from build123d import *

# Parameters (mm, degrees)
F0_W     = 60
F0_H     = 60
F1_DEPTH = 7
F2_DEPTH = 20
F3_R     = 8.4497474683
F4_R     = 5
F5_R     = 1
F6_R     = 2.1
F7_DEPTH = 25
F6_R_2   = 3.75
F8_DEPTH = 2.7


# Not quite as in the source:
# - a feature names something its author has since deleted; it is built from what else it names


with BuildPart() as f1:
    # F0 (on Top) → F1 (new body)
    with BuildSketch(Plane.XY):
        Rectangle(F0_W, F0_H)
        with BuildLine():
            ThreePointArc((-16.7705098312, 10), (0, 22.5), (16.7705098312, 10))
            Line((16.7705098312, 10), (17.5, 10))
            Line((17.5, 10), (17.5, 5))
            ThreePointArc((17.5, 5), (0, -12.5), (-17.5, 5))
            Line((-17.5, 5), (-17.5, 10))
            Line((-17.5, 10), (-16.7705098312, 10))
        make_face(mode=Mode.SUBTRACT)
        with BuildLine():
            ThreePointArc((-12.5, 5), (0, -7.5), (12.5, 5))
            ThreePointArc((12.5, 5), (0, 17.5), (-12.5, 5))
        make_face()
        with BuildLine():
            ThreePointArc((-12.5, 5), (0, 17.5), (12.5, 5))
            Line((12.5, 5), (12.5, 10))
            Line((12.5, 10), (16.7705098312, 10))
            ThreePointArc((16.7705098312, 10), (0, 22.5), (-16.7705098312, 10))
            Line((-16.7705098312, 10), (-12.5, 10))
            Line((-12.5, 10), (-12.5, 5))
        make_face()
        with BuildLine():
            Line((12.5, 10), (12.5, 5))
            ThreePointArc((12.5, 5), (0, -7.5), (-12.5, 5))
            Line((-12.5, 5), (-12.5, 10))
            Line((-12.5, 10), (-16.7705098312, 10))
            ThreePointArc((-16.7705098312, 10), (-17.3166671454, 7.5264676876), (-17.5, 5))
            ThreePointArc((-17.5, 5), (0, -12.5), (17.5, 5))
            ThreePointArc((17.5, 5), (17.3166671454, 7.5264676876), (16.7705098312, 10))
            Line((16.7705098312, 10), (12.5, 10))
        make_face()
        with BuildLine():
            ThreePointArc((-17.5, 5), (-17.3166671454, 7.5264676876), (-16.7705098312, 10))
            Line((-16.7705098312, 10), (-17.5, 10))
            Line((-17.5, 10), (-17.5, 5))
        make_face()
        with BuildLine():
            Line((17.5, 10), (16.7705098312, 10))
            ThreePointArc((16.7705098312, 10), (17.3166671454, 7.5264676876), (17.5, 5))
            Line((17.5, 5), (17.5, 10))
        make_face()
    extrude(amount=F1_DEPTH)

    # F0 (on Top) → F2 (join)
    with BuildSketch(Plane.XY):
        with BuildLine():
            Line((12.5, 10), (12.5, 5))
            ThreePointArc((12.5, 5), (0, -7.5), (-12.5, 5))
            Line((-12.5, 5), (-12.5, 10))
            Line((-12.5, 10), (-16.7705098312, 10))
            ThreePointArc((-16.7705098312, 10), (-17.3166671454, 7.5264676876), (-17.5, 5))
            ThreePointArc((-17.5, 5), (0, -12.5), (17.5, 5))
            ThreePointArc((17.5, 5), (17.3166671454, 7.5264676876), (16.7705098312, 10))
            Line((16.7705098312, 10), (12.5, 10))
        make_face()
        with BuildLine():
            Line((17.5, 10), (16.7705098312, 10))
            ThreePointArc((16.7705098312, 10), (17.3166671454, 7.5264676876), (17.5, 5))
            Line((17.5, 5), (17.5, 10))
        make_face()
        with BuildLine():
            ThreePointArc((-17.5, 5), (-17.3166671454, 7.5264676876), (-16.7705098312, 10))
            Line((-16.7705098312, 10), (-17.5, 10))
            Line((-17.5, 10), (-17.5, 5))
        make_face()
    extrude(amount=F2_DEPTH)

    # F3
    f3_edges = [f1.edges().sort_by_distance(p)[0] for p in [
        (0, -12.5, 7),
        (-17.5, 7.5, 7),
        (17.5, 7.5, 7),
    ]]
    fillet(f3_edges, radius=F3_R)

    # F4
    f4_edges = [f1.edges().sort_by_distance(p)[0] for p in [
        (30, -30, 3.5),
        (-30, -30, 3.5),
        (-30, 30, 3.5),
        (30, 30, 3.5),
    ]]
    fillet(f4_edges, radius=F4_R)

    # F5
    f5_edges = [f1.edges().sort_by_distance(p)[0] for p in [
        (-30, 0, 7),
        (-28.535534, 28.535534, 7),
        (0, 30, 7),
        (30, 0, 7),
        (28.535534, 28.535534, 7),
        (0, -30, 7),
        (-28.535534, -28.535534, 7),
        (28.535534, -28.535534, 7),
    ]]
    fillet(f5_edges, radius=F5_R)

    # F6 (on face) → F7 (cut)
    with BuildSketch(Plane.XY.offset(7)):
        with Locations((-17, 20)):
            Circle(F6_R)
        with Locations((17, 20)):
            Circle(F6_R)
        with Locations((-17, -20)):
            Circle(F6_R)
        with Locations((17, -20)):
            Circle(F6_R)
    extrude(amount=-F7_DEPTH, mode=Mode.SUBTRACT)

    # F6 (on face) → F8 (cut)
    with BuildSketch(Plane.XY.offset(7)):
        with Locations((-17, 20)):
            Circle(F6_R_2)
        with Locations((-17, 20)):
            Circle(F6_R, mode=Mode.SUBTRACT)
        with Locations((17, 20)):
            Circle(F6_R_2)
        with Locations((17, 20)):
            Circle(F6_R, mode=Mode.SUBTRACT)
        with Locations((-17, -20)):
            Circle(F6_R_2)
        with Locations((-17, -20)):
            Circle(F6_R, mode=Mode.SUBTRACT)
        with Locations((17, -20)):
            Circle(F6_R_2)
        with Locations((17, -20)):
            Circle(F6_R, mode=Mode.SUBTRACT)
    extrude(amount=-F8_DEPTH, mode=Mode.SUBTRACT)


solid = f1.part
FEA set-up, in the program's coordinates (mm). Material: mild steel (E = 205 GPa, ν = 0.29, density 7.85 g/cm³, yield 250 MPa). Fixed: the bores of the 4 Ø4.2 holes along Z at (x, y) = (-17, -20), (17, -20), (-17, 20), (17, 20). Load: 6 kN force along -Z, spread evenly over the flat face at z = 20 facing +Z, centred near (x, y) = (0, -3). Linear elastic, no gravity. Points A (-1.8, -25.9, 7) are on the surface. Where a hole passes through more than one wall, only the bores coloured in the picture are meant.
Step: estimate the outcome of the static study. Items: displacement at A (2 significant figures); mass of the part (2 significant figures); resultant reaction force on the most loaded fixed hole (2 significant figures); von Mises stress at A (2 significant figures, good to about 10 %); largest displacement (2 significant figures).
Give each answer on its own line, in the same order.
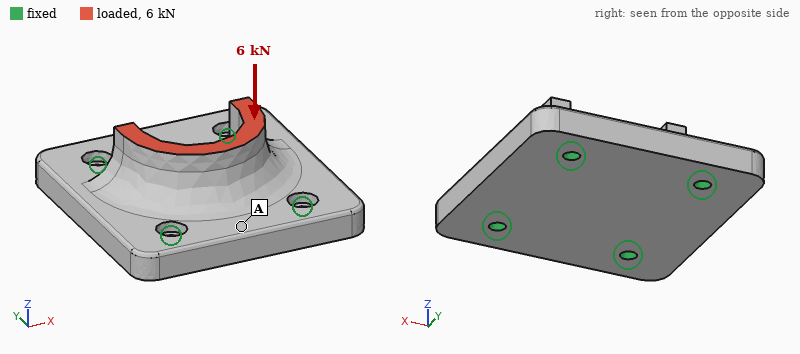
1.9 µm
230 g
2.0 kN
16 MPa
7.7 µm
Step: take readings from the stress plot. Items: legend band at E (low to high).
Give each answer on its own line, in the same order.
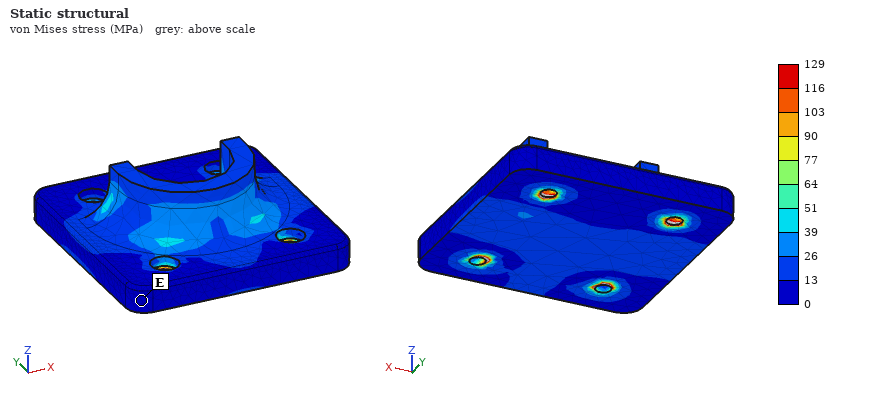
0 to 13 MPa
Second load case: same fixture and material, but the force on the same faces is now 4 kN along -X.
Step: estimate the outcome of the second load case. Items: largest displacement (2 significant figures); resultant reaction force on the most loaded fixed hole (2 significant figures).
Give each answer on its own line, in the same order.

19 µm
2.1 kN
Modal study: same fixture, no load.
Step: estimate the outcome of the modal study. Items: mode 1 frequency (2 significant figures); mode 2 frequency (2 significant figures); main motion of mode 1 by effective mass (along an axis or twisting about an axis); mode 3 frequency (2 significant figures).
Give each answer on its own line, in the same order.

13 kHz
14 kHz
along Z
17 kHz
